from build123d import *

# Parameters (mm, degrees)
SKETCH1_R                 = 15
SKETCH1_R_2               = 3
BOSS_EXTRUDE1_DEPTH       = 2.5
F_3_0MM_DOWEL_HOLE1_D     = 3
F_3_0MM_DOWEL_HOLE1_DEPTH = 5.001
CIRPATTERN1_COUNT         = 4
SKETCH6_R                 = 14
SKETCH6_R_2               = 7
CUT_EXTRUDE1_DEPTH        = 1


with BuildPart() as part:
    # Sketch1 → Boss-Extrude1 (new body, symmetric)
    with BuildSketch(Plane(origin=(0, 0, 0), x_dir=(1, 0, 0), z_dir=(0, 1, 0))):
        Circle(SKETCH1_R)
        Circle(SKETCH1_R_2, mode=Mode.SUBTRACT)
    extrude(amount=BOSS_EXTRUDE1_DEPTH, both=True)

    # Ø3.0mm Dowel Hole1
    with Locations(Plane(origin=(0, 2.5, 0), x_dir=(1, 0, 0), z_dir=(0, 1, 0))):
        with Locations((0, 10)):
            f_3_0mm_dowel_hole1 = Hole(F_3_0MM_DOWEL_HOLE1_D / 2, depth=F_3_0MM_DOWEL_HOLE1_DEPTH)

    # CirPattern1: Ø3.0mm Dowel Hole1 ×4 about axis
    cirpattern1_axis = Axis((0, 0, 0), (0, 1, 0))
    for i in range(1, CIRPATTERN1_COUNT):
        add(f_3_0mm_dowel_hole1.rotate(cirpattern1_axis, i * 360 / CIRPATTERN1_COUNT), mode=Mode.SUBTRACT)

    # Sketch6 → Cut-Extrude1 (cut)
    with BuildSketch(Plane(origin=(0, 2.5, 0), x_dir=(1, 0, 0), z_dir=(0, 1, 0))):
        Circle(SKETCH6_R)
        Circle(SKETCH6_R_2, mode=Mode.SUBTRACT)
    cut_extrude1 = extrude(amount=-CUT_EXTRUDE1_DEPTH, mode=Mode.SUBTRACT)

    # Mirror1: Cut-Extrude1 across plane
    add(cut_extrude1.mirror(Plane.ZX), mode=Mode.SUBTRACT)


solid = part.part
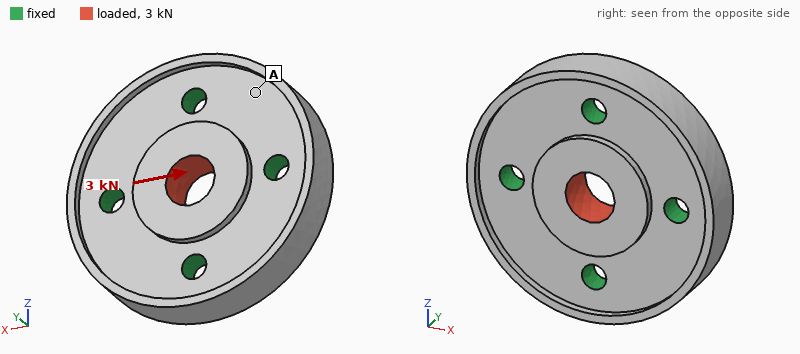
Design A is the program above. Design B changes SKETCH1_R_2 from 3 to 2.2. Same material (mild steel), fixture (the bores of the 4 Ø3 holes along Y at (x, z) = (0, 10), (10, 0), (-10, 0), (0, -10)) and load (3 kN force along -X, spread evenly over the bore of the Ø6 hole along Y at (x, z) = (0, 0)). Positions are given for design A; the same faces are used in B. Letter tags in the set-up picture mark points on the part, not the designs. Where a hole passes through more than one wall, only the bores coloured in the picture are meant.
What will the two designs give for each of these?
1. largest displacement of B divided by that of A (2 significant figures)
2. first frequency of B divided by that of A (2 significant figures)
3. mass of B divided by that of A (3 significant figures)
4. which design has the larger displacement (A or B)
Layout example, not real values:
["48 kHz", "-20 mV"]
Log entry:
["1.1", "1.0", "1.03", "B"]
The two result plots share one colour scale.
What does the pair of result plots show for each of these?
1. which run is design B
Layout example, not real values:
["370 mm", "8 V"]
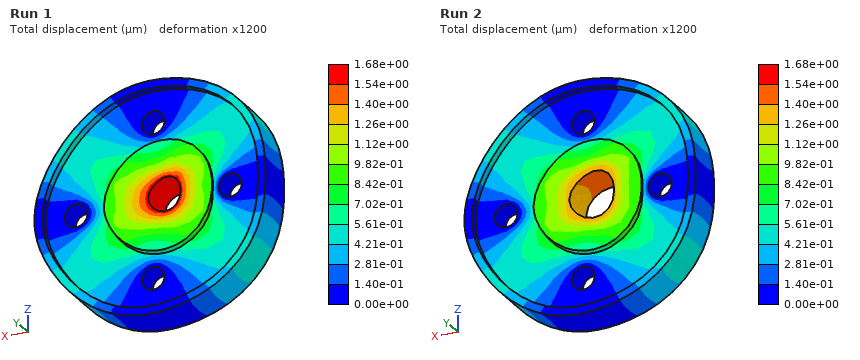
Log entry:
["Run 1"]
